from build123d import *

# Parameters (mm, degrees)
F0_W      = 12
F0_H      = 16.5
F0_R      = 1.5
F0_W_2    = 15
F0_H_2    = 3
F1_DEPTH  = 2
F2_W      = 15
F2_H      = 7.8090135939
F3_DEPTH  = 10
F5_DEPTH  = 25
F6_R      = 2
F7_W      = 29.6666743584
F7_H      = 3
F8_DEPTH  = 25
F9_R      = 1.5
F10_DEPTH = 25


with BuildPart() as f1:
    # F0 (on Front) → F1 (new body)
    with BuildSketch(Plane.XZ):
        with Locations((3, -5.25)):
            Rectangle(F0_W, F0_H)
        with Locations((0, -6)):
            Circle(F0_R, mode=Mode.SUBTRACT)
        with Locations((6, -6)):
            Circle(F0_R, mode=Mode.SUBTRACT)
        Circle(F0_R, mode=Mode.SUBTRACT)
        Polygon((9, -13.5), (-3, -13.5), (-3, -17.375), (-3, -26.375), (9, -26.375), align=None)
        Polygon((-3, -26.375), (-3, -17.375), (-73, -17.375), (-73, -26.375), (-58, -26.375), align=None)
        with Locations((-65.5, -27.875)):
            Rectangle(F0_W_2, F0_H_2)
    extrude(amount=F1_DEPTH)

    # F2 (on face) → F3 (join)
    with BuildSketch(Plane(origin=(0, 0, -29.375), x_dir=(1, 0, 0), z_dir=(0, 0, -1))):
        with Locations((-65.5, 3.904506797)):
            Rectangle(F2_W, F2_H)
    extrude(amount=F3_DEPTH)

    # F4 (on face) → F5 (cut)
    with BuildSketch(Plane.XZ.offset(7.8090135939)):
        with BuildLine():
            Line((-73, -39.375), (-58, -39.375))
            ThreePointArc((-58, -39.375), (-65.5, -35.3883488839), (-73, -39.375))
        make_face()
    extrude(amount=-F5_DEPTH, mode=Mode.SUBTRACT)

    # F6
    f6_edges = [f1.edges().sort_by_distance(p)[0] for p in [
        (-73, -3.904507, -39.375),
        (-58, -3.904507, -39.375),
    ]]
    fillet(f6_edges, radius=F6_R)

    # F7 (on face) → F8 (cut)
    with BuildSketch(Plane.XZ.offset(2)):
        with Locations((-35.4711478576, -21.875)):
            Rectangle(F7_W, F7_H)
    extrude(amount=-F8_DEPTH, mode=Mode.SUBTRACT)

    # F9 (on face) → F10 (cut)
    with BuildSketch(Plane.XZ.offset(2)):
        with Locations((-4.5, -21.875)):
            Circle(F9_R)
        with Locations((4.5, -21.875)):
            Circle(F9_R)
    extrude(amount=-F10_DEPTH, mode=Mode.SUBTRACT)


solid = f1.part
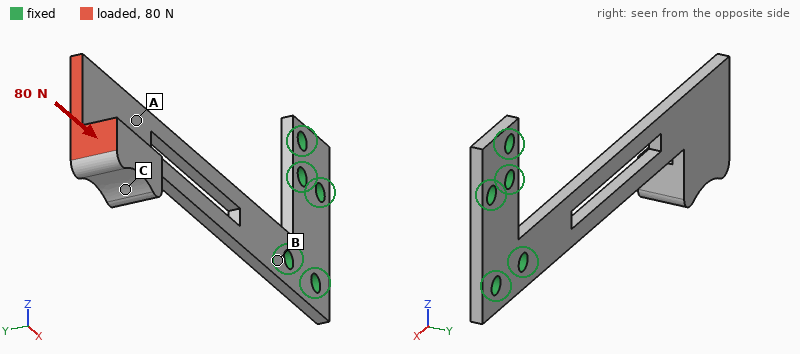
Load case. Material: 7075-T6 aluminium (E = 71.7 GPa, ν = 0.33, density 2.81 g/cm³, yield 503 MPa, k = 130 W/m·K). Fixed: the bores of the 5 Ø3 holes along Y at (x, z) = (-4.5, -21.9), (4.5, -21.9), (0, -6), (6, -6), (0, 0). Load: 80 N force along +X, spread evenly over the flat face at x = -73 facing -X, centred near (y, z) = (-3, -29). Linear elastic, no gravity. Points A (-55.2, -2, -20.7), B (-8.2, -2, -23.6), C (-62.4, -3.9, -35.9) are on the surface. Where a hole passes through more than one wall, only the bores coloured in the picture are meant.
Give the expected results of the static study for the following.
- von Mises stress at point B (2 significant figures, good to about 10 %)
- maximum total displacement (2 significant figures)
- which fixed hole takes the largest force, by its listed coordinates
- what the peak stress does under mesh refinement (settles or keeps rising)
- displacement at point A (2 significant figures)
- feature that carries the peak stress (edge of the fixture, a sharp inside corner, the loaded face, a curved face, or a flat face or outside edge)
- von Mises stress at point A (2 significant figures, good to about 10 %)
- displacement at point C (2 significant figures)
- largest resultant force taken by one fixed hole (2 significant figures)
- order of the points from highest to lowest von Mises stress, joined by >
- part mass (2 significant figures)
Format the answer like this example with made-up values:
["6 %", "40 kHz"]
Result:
["38 MPa", "1.0 mm", "(-4.5, -21.9)", "keeps rising", "0.55 mm", "a sharp inside corner", "22 MPa", "0.74 mm", "79 N", "B > A > C", "7.3 g"]
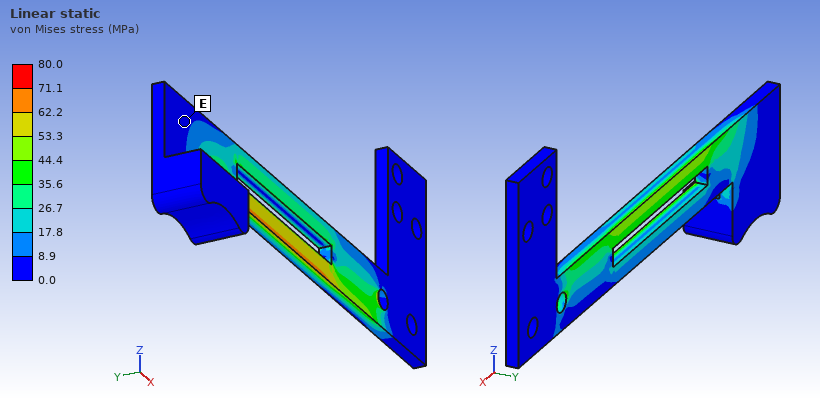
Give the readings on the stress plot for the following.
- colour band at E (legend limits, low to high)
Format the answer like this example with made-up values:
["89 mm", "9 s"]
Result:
["0.0 to 8.9 MPa"]
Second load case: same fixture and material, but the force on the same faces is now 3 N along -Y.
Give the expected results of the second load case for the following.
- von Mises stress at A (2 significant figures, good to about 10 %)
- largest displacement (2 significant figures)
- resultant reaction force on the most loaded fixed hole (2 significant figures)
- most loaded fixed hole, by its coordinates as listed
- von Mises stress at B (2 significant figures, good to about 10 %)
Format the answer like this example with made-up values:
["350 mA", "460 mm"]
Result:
["9.2 MPa", "0.94 mm", "5.6 N", "(-4.5, -21.9)", "31 MPa"]
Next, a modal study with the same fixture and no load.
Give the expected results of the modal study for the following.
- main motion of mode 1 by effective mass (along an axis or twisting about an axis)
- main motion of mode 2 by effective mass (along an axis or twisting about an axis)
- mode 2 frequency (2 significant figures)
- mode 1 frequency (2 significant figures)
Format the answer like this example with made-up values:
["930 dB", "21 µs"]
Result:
["along Y", "along Z", "670 Hz", "180 Hz"]
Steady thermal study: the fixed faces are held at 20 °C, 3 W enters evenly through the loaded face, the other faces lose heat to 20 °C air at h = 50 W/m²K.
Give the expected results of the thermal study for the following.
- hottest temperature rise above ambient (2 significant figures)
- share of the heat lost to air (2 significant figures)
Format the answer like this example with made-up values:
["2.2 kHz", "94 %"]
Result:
["37 K", "73 %"]
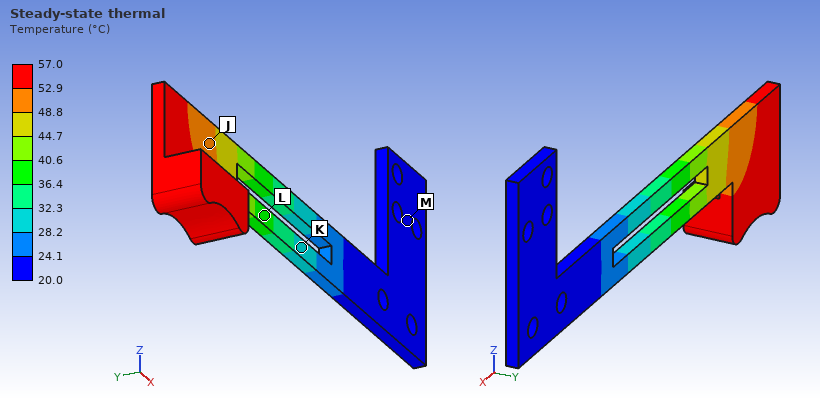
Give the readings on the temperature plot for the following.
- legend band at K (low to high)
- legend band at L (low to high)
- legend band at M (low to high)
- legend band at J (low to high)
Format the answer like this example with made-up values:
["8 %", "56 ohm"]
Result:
["28.2 to 32.3 °C", "36.4 to 40.6 °C", "20.0 to 24.1 °C", "48.8 to 52.9 °C"]
